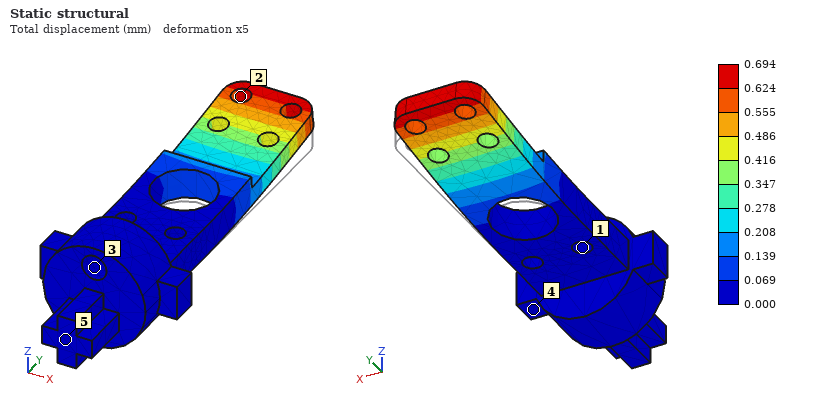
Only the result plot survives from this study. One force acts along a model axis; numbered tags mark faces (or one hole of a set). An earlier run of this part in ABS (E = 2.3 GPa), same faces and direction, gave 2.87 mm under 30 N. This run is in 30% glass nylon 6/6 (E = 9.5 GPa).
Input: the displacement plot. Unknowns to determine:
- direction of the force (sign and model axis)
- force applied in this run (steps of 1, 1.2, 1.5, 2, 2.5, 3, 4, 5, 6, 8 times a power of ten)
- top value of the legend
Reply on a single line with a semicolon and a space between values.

+Z; 30 N; 0.694 mm
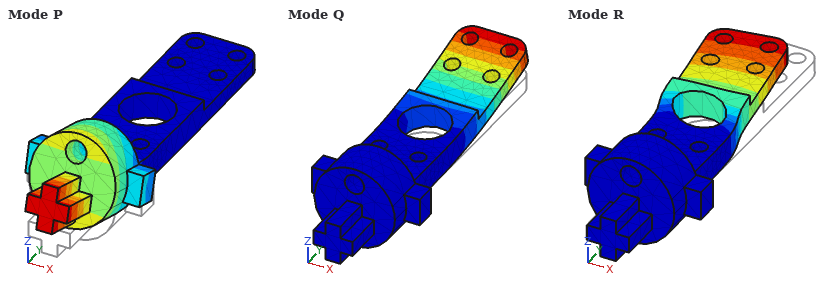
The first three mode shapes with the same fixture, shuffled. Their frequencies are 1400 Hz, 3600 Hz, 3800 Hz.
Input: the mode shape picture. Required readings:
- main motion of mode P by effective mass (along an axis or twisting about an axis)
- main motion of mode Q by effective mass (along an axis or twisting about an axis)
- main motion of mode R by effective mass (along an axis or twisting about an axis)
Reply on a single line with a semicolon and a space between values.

along Z; along Z; along X
